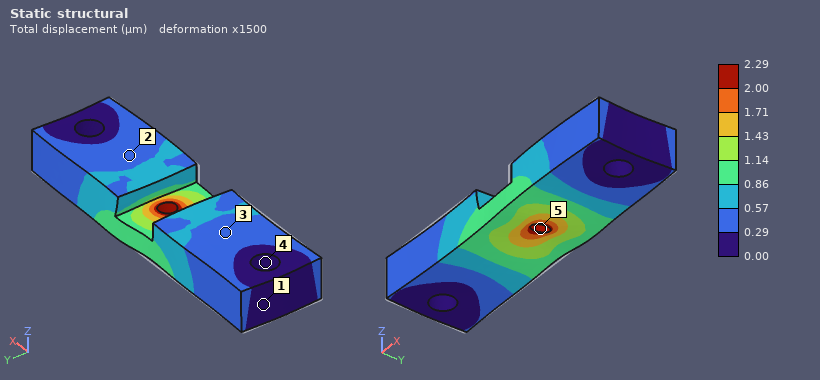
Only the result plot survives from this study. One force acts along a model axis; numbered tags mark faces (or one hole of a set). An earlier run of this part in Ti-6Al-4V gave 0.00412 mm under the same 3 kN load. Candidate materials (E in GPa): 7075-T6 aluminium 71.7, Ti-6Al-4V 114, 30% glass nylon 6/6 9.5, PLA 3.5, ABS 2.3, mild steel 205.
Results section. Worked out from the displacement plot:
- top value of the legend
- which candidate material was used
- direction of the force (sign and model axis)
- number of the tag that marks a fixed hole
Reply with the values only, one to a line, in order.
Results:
2.29 µm
mild steel
+X
4
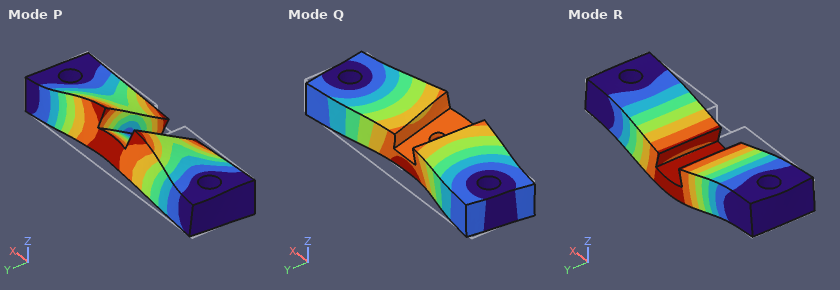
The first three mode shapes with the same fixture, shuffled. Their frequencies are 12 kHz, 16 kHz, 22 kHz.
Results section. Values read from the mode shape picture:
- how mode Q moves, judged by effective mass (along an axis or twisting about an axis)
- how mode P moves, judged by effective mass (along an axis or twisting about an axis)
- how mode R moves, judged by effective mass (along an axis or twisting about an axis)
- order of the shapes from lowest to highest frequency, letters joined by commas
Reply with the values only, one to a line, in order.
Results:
along Y
twisting about X
along Z
R, Q, P
